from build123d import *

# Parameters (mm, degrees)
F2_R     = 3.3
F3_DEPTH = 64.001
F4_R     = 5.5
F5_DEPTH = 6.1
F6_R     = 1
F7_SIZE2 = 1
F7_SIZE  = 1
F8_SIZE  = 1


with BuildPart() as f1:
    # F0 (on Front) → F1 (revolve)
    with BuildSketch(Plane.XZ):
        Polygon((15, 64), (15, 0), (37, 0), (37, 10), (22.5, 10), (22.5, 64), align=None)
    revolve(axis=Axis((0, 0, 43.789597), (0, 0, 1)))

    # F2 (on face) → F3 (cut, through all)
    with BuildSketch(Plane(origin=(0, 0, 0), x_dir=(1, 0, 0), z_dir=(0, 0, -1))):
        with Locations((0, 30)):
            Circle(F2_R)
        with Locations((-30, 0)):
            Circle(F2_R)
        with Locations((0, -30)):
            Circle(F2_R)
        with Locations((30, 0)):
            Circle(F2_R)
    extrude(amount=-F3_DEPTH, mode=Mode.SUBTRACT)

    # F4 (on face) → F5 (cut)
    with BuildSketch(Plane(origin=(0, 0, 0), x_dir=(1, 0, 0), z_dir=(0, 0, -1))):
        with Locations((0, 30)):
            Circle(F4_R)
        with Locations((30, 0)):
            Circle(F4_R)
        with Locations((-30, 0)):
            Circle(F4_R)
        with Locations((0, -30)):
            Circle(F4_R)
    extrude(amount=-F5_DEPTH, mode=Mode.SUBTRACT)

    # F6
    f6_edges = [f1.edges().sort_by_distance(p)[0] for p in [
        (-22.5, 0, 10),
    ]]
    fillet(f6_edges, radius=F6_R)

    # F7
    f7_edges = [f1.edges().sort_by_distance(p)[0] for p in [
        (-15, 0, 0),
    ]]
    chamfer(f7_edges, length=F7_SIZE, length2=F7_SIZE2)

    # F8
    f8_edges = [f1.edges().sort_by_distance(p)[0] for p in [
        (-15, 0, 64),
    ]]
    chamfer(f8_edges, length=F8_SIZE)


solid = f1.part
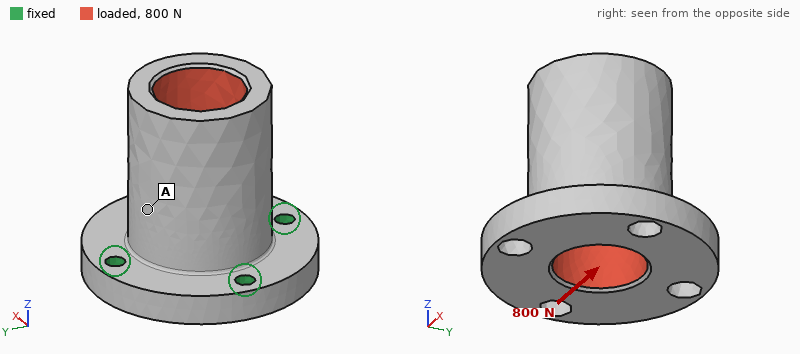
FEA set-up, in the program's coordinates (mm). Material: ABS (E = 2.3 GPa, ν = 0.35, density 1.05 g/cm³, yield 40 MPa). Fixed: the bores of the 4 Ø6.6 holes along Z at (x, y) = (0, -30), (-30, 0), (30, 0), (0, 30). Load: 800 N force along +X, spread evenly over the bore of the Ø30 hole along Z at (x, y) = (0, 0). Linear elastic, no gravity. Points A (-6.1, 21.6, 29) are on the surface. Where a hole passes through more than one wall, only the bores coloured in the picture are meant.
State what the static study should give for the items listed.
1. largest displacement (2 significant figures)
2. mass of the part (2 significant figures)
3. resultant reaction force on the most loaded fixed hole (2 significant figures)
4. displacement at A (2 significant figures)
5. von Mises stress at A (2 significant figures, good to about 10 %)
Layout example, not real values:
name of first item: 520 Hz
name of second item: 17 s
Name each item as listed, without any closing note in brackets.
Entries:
largest displacement: 0.21 mm
mass of the part: 85 g
resultant reaction force on the most loaded fixed hole: 370 N
displacement at A: 0.083 mm
von Mises stress at A: 1.3 MPa
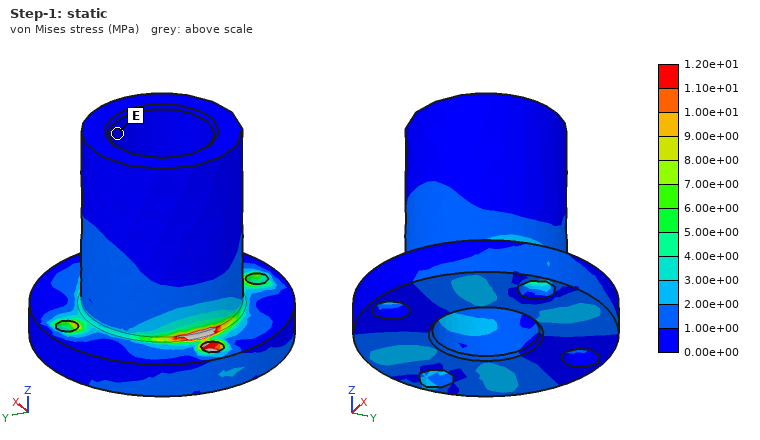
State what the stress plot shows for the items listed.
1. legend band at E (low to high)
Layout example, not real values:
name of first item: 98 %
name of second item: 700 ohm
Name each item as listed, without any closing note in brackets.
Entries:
legend band at E: 0.00e+00 to 1.00e+00 MPa
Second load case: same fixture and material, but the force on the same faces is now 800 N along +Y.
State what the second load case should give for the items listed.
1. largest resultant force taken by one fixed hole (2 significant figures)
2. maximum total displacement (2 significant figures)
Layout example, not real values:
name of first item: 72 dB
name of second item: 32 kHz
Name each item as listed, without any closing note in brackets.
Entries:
largest resultant force taken by one fixed hole: 370 N
maximum total displacement: 0.21 mm
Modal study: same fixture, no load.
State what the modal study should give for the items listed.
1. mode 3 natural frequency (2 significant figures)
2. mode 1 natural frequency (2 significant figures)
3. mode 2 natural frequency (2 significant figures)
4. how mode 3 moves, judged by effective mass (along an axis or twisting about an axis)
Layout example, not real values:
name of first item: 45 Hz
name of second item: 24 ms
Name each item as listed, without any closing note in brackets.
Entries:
mode 3 natural frequency: 2800 Hz
mode 1 natural frequency: 1500 Hz
mode 2 natural frequency: 1500 Hz
how mode 3 moves, judged by effective mass: along Z
